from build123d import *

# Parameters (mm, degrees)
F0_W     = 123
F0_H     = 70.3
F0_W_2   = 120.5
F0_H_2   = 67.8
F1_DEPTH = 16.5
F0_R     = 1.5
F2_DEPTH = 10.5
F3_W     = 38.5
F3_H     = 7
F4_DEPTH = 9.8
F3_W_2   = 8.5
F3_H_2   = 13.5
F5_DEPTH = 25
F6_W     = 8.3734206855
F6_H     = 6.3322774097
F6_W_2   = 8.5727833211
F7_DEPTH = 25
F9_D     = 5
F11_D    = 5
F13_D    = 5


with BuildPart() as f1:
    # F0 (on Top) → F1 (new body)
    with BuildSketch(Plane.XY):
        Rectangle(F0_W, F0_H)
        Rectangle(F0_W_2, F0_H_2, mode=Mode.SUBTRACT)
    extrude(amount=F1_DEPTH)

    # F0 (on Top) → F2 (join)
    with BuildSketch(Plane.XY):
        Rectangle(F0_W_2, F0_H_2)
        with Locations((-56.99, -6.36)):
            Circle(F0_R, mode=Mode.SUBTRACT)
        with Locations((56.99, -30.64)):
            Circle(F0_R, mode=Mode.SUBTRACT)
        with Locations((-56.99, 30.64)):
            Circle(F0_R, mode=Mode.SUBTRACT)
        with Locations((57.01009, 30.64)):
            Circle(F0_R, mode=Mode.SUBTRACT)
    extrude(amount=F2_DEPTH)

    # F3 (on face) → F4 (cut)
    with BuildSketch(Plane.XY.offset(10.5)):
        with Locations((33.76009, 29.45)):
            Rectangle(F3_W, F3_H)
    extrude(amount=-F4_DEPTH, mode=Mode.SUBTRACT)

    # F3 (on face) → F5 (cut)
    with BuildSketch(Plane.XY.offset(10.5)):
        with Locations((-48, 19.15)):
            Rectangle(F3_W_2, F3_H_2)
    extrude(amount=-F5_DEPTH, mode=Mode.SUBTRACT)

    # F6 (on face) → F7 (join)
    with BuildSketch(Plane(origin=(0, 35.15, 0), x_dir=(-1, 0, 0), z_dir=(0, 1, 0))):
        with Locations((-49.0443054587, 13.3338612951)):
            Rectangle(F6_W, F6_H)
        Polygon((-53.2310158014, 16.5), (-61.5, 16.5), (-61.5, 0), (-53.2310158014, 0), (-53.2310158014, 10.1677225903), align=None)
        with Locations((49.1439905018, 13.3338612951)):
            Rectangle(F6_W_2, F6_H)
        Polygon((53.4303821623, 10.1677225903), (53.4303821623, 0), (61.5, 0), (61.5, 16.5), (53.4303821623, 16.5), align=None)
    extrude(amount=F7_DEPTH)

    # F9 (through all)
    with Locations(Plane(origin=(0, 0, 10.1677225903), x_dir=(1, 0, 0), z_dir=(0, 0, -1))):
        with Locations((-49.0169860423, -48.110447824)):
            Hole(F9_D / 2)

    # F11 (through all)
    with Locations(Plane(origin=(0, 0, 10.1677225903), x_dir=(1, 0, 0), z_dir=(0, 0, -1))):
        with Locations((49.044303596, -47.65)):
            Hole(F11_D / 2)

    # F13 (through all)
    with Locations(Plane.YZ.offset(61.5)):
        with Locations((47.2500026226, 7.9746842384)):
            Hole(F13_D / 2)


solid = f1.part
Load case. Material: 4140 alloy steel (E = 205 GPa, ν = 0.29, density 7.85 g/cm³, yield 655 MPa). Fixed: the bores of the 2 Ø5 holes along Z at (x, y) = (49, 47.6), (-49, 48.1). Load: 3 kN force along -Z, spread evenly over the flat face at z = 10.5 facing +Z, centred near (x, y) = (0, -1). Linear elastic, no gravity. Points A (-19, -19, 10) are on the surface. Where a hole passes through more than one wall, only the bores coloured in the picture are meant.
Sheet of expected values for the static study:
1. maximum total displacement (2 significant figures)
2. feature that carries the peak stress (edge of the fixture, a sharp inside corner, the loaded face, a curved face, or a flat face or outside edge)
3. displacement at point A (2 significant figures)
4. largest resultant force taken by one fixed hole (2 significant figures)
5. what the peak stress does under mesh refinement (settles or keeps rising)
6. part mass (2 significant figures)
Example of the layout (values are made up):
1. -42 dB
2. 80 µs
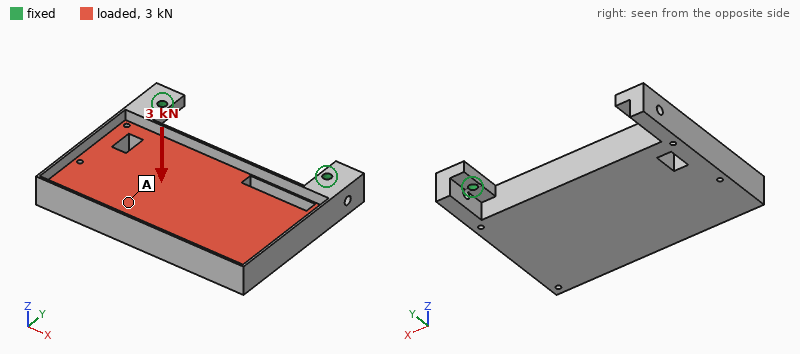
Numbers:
1. 0.60 mm
2. edge of the fixture
3. 0.46 mm
4. 1.6 kN
5. keeps rising
6. 770 g
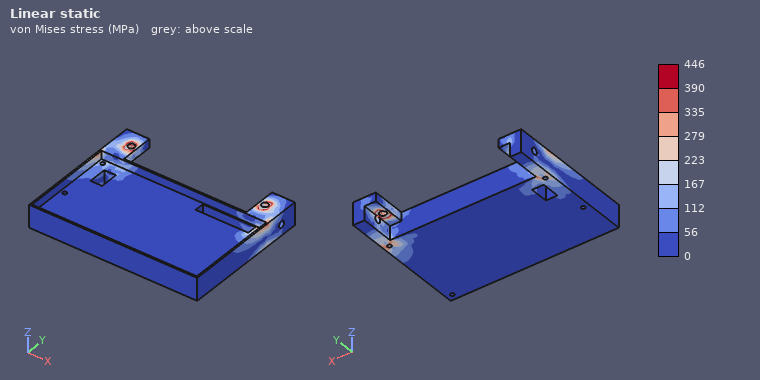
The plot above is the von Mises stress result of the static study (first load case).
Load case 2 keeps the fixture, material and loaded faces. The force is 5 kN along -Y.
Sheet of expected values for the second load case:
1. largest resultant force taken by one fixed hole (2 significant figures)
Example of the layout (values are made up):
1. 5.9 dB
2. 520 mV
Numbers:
1. 2.6 kN
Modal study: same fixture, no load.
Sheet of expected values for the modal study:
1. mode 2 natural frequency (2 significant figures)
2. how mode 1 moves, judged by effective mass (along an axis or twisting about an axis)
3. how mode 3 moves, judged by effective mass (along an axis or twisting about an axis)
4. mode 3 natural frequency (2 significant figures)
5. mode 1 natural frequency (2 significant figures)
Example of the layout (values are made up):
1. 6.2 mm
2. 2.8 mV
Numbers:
1. 1700 Hz
2. along Z
3. along X
4. 2300 Hz
5. 520 Hz
